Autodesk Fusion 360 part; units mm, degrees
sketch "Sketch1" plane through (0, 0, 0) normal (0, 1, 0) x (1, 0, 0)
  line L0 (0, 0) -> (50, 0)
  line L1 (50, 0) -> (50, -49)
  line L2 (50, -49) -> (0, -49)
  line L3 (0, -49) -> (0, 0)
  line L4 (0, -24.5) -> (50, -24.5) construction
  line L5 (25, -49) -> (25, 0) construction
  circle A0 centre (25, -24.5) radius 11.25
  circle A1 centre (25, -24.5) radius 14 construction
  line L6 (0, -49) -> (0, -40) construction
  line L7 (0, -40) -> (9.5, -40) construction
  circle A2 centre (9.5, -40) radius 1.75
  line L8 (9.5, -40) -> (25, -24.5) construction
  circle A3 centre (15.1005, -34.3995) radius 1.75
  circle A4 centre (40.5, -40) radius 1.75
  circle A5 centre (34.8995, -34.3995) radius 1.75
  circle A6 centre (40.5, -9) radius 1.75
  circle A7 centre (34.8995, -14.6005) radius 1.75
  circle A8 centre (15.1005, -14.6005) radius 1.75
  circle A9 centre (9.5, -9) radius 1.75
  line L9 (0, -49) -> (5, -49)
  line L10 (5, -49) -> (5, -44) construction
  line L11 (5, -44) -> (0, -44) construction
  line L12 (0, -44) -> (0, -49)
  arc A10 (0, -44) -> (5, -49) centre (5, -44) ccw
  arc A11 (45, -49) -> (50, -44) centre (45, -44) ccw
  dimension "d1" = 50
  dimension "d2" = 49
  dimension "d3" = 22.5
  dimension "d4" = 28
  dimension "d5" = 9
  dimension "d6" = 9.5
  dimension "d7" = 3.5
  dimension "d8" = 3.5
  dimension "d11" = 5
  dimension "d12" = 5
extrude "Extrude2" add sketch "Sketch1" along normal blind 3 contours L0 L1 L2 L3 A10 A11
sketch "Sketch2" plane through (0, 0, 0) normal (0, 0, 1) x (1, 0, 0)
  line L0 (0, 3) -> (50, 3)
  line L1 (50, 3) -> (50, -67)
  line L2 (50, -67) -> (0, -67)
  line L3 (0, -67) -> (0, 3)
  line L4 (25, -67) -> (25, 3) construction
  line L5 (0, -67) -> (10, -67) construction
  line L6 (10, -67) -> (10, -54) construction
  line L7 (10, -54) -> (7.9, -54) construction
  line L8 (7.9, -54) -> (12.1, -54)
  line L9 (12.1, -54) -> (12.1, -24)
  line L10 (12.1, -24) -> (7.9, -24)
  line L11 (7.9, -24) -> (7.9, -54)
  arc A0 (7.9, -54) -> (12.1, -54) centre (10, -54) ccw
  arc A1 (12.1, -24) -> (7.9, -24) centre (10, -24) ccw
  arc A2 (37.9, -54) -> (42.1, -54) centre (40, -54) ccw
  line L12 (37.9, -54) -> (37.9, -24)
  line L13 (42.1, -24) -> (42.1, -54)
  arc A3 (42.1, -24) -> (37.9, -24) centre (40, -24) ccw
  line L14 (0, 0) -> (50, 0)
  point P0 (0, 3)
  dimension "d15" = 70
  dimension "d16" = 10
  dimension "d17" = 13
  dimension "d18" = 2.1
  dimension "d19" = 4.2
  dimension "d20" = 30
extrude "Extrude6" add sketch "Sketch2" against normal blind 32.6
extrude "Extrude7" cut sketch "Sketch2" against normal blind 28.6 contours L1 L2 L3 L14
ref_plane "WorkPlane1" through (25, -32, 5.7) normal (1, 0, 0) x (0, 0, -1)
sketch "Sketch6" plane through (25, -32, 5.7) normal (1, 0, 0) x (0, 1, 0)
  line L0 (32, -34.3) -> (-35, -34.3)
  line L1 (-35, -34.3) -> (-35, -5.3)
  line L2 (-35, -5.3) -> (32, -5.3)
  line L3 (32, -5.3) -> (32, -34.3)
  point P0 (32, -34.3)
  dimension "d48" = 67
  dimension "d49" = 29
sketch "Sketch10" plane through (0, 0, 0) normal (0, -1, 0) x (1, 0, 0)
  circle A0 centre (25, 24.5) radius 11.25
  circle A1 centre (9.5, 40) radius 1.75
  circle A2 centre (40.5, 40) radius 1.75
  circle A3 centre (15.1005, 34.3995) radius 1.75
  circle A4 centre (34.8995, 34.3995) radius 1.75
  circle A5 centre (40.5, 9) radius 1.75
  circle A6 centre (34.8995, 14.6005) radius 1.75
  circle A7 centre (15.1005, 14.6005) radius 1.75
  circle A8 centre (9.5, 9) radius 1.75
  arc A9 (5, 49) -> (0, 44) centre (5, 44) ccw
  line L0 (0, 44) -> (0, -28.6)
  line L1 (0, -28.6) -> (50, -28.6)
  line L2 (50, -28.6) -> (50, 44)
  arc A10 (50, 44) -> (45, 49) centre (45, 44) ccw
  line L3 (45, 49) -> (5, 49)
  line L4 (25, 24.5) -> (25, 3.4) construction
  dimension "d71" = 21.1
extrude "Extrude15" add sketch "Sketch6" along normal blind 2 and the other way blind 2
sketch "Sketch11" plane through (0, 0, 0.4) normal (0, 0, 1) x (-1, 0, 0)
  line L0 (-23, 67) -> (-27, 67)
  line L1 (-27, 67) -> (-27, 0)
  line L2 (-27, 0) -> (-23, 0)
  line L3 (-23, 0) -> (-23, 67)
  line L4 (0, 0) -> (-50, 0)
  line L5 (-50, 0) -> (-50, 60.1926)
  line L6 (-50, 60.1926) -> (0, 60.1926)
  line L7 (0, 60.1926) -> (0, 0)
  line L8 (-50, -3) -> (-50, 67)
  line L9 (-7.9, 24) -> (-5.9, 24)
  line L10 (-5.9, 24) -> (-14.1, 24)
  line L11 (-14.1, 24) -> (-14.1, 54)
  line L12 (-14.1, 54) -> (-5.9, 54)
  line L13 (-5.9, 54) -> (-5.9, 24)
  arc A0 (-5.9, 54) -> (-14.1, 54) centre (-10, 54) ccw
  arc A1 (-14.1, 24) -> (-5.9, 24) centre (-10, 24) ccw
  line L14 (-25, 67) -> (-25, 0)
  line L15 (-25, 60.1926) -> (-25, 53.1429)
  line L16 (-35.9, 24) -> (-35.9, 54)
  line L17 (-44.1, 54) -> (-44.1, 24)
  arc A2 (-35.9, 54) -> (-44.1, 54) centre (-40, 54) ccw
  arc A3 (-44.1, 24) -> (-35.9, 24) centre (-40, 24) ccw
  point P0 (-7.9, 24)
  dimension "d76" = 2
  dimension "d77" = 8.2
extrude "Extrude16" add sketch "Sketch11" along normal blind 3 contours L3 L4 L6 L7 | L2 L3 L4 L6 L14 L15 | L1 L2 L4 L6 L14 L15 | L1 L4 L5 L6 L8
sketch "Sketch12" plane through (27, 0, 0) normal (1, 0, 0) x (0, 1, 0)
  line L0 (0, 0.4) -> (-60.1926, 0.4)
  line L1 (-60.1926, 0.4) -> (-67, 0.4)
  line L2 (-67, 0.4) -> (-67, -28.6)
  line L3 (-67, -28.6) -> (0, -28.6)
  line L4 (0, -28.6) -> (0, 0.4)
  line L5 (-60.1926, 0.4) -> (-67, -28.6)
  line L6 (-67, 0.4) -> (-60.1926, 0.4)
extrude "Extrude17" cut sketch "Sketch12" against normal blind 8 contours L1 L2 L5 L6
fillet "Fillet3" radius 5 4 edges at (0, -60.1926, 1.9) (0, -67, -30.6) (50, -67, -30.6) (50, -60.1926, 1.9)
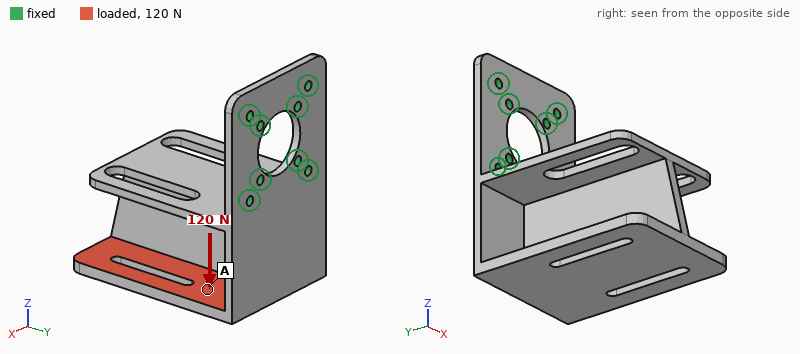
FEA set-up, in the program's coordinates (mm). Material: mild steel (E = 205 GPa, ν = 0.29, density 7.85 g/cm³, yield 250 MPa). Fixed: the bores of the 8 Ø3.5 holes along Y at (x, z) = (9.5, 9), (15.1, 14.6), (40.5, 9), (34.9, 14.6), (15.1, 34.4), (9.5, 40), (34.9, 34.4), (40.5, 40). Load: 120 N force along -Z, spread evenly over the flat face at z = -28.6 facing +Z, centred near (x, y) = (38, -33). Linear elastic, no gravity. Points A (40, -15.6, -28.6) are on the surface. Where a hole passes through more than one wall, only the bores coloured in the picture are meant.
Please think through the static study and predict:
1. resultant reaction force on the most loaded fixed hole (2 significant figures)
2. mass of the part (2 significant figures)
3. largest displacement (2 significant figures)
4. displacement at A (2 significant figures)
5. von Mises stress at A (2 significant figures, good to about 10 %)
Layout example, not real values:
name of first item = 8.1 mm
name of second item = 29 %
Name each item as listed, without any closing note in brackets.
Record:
resultant reaction force on the most loaded fixed hole = 140 N
mass of the part = 300 g
largest displacement = 0.13 mm
displacement at A = 0.059 mm
von Mises stress at A = 5.9 MPa
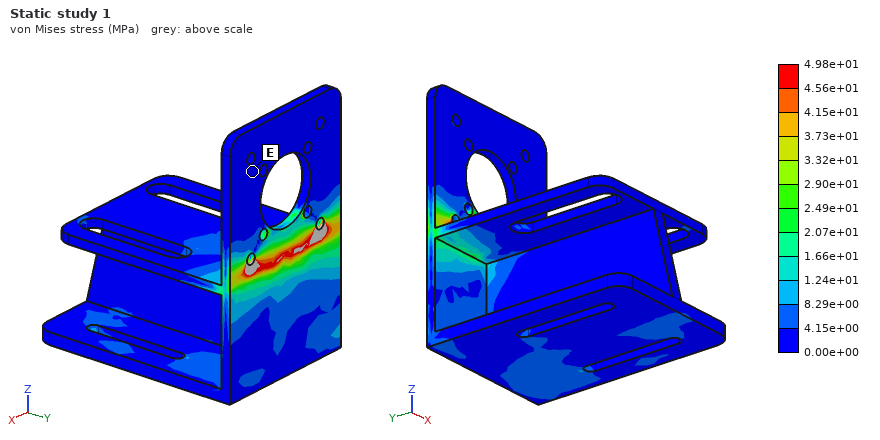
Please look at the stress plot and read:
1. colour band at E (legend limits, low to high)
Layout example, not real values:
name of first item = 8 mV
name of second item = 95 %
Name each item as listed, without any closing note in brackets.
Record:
colour band at E = 0.00e+00 to 4.15e+00 MPa
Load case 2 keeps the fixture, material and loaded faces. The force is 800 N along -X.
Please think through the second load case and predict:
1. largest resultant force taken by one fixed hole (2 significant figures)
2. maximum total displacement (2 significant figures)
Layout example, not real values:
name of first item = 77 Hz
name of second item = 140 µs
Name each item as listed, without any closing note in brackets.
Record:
largest resultant force taken by one fixed hole = 1.2 kN
maximum total displacement = 0.22 mm
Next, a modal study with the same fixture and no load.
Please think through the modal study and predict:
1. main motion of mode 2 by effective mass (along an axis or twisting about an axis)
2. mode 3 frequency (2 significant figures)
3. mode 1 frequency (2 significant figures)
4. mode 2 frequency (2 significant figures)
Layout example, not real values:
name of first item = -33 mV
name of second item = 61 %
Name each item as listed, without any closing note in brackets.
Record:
main motion of mode 2 by effective mass = along X
mode 3 frequency = 2800 Hz
mode 1 frequency = 380 Hz
mode 2 frequency = 1000 Hz
